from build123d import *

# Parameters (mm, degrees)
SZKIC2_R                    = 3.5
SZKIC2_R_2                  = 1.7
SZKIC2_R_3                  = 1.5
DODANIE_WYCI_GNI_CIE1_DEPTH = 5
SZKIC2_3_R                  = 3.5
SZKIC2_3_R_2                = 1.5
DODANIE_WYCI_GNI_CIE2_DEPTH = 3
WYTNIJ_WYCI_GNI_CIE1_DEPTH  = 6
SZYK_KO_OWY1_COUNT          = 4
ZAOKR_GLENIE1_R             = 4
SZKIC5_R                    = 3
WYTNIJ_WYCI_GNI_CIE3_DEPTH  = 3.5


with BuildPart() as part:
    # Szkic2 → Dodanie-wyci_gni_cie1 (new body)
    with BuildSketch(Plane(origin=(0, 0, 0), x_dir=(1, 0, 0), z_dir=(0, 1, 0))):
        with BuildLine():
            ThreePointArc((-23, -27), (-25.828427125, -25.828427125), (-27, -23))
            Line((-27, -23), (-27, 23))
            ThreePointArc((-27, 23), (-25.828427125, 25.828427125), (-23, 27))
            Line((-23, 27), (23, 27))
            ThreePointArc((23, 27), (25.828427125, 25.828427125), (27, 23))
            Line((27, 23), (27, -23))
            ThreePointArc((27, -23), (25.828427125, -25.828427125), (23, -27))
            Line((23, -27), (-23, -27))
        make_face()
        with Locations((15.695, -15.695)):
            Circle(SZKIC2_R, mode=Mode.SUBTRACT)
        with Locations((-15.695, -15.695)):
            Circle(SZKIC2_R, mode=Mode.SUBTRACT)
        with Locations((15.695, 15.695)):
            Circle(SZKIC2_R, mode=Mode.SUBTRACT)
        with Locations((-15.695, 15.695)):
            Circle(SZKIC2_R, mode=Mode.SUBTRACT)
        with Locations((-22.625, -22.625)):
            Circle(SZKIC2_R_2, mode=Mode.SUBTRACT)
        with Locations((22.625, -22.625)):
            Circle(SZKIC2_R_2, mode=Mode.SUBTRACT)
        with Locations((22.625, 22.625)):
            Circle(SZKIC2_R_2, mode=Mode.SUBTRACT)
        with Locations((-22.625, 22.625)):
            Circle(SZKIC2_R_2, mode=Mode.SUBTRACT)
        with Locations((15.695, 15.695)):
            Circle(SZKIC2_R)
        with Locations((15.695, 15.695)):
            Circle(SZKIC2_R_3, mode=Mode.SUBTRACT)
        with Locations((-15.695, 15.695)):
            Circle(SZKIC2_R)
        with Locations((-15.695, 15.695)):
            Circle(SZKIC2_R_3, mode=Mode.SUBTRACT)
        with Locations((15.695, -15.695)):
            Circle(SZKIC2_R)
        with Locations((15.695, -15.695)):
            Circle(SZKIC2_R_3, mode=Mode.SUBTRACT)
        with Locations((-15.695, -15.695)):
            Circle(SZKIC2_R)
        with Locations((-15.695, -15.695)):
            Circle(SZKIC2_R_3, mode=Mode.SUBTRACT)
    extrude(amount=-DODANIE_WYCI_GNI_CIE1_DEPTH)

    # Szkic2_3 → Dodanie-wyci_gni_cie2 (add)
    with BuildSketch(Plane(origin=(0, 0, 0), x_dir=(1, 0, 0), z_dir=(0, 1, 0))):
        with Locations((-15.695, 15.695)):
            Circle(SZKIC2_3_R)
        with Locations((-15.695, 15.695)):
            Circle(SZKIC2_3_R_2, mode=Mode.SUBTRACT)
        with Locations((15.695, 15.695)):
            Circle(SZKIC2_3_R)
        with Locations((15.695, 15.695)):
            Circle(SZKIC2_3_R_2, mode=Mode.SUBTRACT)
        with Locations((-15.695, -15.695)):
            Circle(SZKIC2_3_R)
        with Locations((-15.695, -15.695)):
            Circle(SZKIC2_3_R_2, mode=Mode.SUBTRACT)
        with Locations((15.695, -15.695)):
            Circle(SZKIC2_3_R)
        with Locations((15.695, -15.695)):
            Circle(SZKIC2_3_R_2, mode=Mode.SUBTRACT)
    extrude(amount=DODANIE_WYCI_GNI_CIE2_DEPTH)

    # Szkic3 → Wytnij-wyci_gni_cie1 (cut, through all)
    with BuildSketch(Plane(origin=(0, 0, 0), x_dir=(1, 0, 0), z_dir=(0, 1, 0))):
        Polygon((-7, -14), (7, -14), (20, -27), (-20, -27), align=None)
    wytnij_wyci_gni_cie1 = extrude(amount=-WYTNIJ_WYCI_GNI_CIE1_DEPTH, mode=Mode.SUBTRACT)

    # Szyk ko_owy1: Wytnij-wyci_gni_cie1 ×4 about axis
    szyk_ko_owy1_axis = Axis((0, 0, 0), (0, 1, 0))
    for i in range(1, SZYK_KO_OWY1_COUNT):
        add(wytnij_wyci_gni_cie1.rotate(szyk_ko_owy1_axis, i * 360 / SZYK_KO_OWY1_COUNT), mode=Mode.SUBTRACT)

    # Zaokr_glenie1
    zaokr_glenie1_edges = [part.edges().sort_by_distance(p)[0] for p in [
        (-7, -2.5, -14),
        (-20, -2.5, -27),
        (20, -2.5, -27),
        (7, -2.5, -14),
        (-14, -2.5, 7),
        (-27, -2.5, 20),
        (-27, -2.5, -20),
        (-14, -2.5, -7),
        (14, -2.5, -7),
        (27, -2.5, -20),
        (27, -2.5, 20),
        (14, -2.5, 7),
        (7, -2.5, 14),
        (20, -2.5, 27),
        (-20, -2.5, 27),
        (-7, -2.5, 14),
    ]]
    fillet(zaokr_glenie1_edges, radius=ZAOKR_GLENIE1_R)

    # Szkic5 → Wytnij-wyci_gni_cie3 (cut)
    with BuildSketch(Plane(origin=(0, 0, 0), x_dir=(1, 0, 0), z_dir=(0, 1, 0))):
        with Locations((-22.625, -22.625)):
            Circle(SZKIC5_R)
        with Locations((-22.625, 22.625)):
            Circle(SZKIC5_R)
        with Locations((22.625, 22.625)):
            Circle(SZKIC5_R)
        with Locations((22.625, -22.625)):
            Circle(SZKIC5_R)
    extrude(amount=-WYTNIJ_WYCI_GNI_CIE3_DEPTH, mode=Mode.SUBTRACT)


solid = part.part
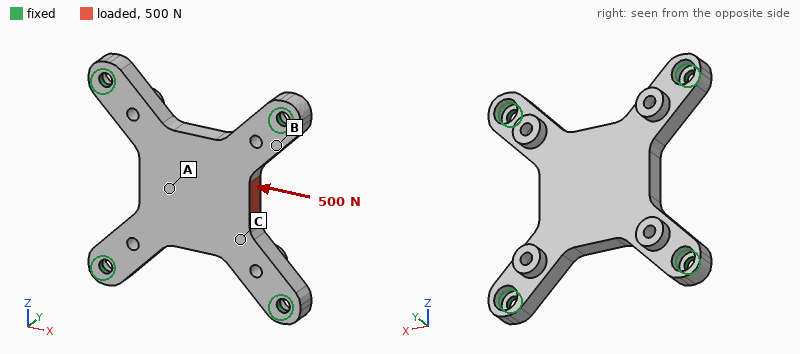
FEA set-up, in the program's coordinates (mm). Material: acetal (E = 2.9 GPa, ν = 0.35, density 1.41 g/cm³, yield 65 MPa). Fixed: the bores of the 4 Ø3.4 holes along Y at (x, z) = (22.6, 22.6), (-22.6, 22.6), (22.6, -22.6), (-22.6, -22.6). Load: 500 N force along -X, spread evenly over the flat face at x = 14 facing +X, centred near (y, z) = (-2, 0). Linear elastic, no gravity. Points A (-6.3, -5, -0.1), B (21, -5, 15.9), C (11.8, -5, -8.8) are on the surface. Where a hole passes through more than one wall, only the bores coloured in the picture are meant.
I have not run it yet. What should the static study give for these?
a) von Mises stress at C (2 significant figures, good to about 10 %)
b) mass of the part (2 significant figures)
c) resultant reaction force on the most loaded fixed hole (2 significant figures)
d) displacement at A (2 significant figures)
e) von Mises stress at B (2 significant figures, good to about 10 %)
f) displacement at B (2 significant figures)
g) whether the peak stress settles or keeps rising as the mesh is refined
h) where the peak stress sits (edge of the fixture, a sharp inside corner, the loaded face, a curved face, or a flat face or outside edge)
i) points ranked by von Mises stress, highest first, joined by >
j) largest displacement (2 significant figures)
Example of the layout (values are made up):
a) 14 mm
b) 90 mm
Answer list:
a) 3.8 MPa
b) 10 g
c) 160 N
d) 0.072 mm
e) 7.7 MPa
f) 0.040 mm
g) keeps rising
h) edge of the fixture
i) B > C > A
j) 0.12 mm
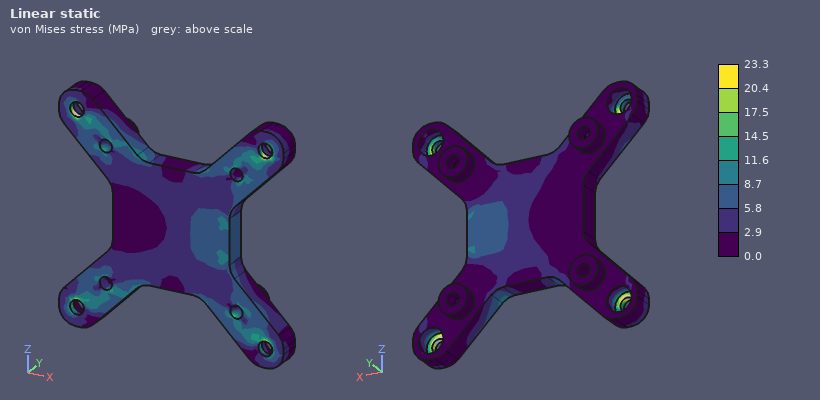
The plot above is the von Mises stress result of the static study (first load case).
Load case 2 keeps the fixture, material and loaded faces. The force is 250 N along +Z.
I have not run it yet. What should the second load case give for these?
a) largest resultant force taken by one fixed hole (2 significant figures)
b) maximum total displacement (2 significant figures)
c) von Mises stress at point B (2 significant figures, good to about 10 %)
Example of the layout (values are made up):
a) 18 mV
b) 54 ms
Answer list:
a) 93 N
b) 78 µm
c) 5.7 MPa
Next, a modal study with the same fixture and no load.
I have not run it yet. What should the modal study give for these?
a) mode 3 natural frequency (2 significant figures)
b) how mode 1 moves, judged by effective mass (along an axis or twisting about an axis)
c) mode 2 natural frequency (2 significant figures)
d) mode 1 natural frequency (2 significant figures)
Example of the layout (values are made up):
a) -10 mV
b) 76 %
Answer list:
a) 3400 Hz
b) along Y
c) 3400 Hz
d) 1600 Hz
